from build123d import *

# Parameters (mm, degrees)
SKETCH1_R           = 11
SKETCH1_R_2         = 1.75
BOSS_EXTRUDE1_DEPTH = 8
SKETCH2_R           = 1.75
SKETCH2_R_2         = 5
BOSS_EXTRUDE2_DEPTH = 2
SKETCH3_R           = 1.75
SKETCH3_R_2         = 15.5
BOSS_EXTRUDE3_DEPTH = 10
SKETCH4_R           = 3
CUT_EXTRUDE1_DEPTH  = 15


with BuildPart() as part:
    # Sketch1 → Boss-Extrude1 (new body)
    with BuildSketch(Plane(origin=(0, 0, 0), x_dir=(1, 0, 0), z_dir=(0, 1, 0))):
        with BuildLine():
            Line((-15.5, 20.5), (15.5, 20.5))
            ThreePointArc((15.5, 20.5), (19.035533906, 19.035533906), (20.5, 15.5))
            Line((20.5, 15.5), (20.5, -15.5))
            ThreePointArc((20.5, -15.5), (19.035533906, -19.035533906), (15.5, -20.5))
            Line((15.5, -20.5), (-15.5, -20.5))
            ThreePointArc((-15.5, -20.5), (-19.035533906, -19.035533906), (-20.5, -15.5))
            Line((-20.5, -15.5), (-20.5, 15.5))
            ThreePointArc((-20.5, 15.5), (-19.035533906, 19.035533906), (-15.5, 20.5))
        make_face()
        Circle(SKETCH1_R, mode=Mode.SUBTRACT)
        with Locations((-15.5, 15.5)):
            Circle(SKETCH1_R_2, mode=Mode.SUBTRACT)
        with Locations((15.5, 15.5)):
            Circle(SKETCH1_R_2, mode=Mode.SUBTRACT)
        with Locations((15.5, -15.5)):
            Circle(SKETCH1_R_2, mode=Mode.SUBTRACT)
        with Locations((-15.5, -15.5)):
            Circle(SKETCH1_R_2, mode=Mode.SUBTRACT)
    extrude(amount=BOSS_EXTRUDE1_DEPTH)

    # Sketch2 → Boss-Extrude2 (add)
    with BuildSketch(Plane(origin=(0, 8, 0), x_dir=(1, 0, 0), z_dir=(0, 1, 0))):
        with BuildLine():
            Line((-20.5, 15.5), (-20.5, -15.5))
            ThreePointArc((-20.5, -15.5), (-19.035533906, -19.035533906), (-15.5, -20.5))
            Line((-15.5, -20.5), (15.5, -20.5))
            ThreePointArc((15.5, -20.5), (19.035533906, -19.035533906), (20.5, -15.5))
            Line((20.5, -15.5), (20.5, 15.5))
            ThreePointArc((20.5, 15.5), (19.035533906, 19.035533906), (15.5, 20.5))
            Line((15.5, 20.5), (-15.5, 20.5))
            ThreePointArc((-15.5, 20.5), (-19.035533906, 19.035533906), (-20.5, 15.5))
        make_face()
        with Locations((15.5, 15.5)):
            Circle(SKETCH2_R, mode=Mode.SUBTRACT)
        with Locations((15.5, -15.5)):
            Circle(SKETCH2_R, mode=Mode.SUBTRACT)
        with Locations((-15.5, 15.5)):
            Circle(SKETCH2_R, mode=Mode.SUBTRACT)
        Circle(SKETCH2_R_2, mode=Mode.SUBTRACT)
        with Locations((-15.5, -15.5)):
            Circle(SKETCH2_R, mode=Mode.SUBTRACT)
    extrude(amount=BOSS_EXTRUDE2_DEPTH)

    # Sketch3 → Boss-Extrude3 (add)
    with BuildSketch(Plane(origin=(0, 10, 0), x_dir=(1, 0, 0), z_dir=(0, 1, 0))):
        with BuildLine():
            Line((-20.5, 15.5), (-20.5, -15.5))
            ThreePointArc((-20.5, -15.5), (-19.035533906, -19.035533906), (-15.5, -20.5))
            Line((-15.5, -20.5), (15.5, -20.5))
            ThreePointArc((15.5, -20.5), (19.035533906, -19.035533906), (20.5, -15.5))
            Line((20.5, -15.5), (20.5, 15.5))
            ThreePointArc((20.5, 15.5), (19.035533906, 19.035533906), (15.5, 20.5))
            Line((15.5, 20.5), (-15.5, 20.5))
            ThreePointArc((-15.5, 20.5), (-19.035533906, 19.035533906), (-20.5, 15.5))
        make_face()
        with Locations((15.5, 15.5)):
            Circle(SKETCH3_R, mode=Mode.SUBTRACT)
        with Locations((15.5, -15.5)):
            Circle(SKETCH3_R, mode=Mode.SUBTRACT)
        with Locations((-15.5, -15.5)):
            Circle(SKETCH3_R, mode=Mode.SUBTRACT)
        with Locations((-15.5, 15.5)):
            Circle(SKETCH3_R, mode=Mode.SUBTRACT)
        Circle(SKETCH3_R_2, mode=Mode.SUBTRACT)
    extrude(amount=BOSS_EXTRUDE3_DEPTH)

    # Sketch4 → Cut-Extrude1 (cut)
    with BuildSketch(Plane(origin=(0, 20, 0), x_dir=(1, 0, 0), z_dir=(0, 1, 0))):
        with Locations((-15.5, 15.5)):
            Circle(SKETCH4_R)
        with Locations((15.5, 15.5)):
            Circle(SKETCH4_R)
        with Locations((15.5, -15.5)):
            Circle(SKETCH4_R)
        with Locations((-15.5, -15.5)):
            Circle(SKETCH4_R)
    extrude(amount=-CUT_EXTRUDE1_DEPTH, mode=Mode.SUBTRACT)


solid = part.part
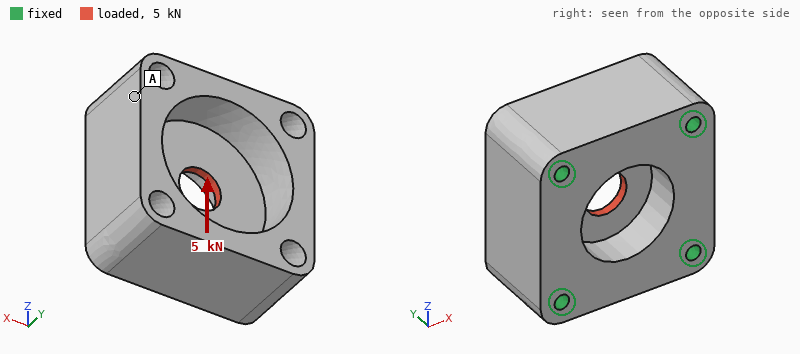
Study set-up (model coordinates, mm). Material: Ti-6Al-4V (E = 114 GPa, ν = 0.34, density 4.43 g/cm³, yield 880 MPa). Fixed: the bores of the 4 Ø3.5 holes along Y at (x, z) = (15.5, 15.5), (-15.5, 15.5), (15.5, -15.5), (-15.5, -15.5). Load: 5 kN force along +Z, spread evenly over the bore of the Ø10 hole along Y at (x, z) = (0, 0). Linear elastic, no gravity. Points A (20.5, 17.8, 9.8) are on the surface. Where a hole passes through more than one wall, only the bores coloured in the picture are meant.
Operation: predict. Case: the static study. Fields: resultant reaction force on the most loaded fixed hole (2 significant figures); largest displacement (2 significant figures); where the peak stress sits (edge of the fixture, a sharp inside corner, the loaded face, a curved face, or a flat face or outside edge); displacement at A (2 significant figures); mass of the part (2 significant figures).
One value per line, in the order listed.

1.4 kN
9.7 µm
the loaded face
1.9 µm
91 g
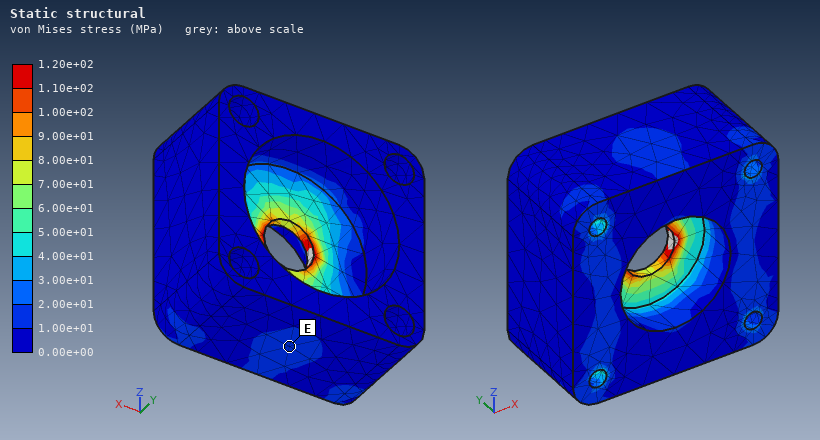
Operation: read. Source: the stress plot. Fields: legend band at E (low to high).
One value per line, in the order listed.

1.00e+01 to 2.00e+01 MPa
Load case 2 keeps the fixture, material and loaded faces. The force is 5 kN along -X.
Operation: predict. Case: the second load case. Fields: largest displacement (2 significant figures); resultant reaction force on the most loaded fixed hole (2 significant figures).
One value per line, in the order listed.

9.7 µm
1.4 kN
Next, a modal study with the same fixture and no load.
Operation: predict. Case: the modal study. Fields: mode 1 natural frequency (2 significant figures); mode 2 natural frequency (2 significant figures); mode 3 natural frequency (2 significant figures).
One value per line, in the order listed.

21 kHz
23 kHz
23 kHz
